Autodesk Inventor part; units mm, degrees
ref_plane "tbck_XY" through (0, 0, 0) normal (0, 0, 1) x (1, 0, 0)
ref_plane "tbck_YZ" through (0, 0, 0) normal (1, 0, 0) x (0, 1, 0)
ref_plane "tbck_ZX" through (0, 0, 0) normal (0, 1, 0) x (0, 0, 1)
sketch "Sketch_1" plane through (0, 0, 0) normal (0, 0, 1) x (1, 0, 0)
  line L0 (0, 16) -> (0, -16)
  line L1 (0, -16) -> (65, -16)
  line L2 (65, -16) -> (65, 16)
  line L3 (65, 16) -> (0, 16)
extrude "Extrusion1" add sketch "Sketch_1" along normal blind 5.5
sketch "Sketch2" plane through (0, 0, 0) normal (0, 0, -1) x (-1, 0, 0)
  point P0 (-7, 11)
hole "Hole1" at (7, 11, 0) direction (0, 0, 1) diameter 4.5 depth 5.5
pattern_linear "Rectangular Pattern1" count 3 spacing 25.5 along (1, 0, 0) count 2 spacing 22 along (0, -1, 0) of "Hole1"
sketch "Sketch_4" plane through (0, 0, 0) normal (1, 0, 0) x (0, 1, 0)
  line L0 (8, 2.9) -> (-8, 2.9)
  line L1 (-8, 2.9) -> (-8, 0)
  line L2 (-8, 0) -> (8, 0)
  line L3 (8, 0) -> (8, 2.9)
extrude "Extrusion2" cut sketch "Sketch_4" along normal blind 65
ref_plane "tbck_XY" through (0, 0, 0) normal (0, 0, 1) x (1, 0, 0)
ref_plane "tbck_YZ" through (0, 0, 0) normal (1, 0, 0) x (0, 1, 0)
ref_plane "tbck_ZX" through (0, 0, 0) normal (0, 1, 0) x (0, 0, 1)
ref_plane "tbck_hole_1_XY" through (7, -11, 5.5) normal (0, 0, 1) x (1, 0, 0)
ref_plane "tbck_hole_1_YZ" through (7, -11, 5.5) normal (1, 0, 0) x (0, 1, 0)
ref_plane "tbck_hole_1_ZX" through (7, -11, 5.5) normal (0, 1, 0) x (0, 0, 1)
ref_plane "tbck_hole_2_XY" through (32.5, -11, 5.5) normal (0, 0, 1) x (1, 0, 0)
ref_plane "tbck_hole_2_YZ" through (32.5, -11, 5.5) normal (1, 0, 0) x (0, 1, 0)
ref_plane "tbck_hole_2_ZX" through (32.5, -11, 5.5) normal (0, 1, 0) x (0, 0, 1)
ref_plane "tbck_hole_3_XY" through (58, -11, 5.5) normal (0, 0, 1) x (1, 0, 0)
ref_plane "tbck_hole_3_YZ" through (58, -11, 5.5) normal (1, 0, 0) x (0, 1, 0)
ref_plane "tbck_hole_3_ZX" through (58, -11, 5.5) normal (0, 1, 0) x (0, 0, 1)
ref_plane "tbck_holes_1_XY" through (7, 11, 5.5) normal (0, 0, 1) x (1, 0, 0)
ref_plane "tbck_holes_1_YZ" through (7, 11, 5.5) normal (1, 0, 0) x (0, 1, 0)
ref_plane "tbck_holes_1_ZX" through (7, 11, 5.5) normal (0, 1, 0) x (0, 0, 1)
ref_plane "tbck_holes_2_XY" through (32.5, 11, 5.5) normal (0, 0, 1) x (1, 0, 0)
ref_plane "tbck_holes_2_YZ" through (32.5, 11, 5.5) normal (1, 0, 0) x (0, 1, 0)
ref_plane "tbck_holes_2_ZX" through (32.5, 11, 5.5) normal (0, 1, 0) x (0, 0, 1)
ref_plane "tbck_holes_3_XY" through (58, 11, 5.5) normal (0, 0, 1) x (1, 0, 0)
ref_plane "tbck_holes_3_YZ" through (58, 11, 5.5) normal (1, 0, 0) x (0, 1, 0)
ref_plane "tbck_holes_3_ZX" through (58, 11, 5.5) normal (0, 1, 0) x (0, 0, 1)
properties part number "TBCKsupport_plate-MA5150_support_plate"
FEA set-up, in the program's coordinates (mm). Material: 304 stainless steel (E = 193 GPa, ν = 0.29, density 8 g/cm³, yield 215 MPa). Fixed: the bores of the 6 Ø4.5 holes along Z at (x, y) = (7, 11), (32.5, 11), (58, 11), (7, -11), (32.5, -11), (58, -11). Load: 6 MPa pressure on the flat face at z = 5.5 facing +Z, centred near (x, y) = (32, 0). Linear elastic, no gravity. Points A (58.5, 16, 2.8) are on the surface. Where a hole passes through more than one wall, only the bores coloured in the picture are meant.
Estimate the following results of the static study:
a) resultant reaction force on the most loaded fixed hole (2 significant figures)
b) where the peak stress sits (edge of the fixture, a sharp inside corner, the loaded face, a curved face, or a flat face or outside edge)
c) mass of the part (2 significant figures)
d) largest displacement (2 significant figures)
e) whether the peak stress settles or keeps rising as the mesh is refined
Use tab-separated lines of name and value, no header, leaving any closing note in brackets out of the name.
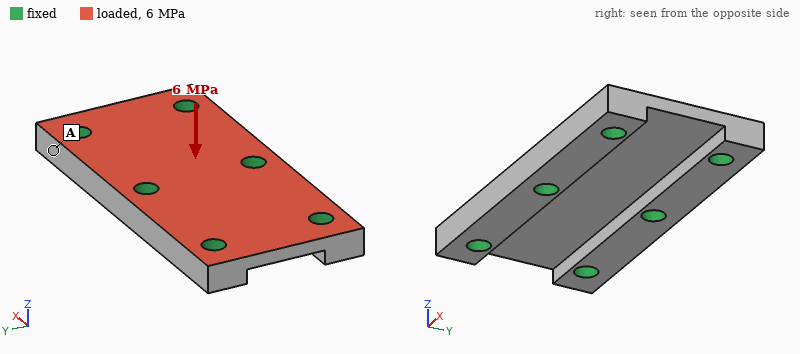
resultant reaction force on the most loaded fixed hole	2.4 kN
where the peak stress sits	edge of the fixture
mass of the part	63 g
largest displacement	13 µm
whether the peak stress settles or keeps rising as the mesh is refined	keeps rising
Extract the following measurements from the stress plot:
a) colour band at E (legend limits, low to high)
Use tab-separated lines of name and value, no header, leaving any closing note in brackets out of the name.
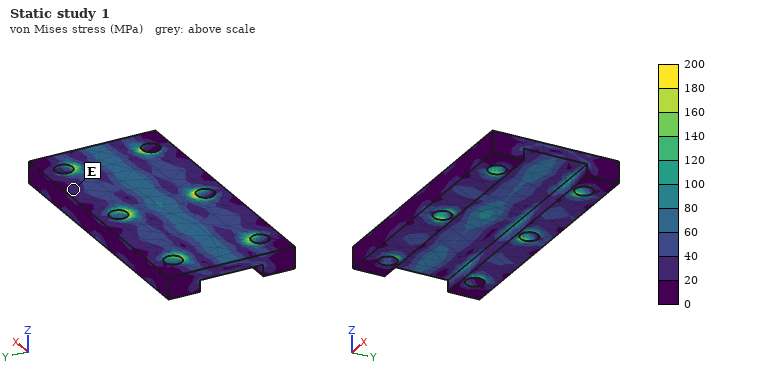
colour band at E	20 to 40 MPa
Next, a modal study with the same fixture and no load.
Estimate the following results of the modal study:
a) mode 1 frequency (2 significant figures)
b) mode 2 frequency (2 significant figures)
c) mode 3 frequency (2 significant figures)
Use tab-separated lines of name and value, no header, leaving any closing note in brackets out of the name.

mode 1 frequency	28 kHz
mode 2 frequency	28 kHz
mode 3 frequency	37 kHz
